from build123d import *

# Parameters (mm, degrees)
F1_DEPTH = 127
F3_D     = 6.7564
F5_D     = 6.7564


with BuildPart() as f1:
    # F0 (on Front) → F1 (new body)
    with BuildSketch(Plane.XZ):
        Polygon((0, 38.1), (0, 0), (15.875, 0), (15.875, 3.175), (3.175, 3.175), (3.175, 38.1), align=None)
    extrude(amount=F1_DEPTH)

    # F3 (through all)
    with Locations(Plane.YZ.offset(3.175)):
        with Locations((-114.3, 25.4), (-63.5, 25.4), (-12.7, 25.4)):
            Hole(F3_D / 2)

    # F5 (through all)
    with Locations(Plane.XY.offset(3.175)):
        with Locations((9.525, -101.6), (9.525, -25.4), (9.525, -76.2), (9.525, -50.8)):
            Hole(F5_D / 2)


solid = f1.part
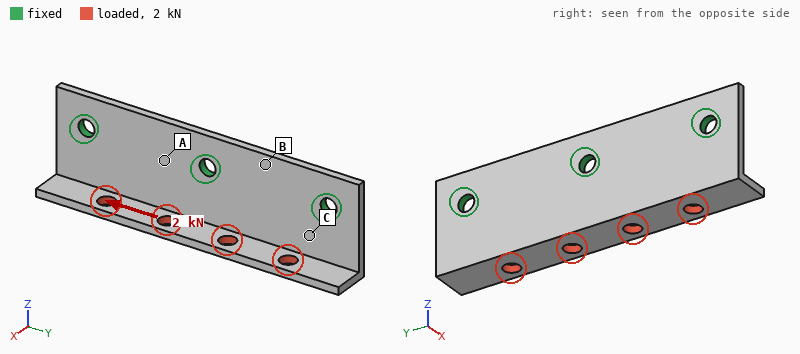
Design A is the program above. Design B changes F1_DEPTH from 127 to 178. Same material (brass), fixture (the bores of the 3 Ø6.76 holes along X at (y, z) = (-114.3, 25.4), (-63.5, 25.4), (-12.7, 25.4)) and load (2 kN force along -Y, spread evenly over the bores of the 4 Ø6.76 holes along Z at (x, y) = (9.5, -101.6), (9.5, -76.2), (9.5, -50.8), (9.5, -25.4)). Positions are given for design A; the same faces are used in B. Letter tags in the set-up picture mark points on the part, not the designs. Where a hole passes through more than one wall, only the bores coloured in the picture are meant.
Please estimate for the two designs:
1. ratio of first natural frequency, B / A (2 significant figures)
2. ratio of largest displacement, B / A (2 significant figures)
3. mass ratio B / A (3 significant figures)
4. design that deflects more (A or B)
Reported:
0.49
1.2
1.42
B
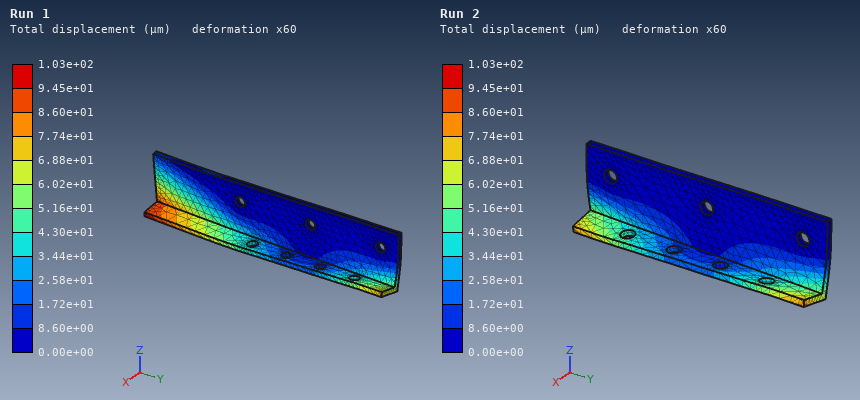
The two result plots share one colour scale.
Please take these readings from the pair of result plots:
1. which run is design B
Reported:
Run 1
